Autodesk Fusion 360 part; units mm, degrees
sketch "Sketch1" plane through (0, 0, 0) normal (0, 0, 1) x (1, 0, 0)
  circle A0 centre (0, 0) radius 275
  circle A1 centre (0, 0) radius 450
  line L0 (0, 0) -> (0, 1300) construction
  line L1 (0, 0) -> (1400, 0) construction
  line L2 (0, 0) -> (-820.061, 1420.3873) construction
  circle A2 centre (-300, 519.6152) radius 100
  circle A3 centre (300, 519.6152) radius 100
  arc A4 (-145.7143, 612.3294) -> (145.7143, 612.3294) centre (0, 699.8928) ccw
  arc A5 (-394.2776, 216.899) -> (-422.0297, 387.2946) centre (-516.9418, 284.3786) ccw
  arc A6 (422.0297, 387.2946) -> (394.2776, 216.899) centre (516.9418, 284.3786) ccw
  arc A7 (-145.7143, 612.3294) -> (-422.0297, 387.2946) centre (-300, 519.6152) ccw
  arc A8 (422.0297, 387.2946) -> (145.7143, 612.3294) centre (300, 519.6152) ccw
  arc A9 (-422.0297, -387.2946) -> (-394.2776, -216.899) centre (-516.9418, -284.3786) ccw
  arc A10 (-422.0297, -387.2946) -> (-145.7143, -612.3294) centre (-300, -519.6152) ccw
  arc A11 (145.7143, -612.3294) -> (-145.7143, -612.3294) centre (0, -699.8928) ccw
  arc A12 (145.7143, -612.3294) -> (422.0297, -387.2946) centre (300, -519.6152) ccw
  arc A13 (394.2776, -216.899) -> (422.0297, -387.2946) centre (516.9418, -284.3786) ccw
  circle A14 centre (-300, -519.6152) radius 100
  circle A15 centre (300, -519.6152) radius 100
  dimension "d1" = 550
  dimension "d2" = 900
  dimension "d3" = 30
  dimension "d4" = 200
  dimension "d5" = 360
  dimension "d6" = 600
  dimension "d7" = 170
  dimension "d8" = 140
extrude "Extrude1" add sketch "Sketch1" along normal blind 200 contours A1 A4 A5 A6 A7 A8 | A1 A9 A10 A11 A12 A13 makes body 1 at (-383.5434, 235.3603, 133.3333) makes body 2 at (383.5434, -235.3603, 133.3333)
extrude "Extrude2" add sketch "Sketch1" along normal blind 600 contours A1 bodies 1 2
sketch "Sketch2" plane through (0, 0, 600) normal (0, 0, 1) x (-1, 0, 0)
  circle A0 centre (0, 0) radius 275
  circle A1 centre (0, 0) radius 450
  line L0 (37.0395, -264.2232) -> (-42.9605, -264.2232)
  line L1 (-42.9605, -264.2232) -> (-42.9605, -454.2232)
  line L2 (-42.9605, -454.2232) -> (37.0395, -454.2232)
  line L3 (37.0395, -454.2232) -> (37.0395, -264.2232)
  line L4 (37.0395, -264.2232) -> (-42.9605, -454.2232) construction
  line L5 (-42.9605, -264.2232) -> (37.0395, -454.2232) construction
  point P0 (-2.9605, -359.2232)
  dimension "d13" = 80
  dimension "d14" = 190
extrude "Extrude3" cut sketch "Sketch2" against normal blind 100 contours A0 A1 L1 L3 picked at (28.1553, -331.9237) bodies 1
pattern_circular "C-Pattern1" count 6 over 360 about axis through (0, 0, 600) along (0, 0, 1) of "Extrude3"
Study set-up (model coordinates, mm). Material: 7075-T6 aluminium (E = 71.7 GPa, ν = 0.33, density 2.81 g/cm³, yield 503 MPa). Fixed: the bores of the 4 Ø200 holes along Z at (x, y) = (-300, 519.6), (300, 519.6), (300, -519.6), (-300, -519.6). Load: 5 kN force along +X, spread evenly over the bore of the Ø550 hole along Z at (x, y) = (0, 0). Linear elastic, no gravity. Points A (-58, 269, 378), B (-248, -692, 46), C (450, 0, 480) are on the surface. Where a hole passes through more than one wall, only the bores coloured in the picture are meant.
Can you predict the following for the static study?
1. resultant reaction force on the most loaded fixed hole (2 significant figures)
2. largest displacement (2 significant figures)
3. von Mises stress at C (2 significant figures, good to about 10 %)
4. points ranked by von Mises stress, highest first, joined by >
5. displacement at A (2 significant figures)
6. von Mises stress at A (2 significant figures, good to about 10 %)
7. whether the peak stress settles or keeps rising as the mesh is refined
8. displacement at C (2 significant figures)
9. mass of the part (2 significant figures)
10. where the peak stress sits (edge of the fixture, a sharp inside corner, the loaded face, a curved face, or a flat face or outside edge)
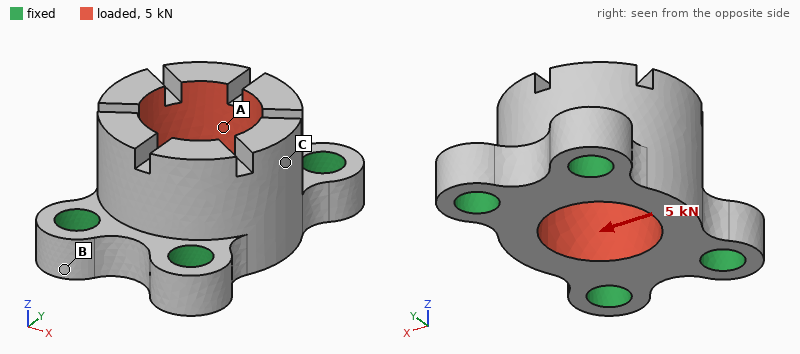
1.6 kN
0.60 µm
0.015 MPa
A > C > B
0.27 µm
0.028 MPa
keeps rising
0.50 µm
840 kg
edge of the fixture
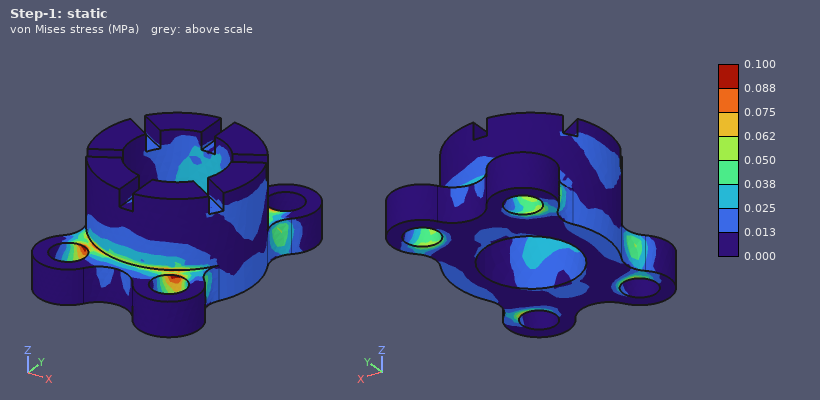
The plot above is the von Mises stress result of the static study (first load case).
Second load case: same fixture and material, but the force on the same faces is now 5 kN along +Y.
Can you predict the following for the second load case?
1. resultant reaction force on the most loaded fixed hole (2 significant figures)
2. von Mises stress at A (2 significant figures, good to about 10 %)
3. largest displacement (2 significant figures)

1.4 kN
0.0087 MPa
0.33 µm
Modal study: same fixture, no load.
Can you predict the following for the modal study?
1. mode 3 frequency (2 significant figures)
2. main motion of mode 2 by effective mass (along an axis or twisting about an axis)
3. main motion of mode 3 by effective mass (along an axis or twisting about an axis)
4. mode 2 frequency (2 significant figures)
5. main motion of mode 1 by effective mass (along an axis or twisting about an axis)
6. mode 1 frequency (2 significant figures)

1000 Hz
along Z
along Y
770 Hz
along X
670 Hz
